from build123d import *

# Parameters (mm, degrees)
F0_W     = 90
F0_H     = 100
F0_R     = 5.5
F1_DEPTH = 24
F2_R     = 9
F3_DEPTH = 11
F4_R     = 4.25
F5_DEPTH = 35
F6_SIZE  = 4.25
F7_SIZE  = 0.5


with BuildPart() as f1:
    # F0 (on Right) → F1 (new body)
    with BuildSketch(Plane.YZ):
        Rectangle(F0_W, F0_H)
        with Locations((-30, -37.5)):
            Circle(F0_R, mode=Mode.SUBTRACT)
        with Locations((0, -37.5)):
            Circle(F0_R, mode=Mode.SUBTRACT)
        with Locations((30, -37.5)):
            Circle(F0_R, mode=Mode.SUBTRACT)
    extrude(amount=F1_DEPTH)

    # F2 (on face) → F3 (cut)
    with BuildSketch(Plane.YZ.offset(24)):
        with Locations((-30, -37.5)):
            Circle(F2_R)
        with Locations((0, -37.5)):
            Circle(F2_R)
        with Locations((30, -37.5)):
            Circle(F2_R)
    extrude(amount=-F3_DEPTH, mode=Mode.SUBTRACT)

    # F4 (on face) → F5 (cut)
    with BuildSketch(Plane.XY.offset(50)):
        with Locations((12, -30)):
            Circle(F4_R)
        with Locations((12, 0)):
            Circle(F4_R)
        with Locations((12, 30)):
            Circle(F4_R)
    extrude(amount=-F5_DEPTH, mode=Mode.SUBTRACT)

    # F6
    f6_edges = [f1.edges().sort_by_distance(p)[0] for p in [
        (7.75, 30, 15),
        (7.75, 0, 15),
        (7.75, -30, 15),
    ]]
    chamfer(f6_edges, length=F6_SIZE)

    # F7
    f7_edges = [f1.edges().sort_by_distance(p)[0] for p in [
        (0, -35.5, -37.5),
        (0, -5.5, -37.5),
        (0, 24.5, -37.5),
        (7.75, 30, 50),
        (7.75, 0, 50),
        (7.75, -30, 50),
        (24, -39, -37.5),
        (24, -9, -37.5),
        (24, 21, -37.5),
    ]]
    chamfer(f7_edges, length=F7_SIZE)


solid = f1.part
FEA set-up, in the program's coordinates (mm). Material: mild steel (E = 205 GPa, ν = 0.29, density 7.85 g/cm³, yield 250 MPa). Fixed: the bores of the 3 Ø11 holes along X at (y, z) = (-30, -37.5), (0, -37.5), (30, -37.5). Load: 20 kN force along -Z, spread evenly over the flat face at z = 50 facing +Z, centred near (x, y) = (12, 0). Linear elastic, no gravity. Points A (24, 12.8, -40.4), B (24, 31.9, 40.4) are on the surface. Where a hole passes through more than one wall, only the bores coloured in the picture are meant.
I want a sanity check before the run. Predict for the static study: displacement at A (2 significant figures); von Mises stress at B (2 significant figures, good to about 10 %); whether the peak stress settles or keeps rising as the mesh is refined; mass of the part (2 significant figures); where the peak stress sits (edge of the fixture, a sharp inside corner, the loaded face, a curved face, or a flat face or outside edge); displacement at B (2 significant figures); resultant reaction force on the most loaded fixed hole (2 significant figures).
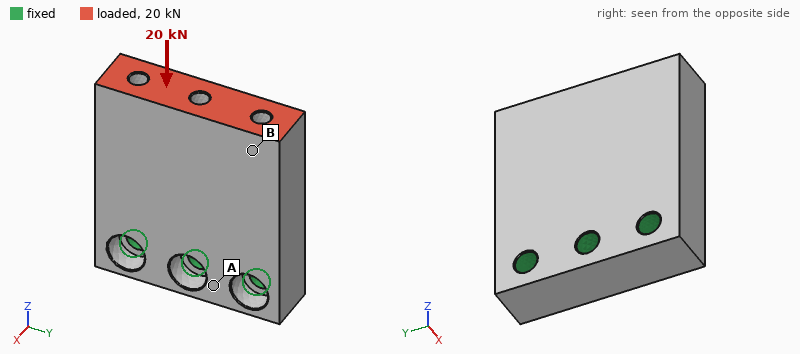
2.7 µm
10 MPa
keeps rising
1.6 kg
edge of the fixture
14 µm
6.8 kN
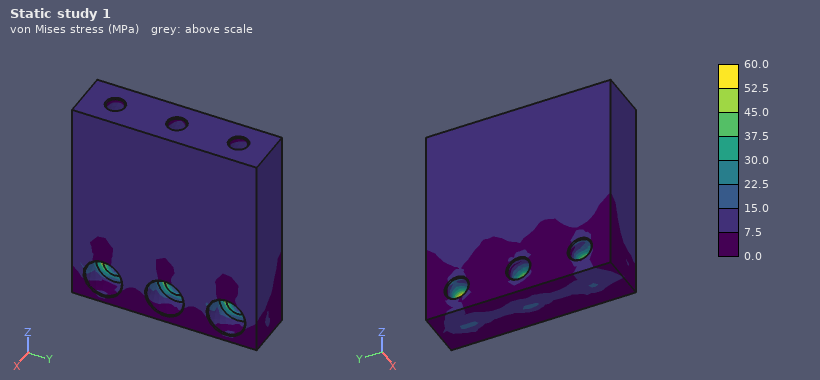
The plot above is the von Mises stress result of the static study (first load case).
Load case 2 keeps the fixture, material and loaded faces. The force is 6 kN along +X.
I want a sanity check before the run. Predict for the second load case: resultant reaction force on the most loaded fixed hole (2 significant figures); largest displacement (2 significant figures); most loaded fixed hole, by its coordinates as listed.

3.2 kN
0.11 mm
(0, -37.5)
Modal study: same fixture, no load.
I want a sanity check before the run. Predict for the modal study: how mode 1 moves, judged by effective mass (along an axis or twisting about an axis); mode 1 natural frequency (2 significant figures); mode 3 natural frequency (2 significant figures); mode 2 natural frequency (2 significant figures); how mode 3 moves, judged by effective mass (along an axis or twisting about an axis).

along X
1900 Hz
5600 Hz
4600 Hz
along Y
